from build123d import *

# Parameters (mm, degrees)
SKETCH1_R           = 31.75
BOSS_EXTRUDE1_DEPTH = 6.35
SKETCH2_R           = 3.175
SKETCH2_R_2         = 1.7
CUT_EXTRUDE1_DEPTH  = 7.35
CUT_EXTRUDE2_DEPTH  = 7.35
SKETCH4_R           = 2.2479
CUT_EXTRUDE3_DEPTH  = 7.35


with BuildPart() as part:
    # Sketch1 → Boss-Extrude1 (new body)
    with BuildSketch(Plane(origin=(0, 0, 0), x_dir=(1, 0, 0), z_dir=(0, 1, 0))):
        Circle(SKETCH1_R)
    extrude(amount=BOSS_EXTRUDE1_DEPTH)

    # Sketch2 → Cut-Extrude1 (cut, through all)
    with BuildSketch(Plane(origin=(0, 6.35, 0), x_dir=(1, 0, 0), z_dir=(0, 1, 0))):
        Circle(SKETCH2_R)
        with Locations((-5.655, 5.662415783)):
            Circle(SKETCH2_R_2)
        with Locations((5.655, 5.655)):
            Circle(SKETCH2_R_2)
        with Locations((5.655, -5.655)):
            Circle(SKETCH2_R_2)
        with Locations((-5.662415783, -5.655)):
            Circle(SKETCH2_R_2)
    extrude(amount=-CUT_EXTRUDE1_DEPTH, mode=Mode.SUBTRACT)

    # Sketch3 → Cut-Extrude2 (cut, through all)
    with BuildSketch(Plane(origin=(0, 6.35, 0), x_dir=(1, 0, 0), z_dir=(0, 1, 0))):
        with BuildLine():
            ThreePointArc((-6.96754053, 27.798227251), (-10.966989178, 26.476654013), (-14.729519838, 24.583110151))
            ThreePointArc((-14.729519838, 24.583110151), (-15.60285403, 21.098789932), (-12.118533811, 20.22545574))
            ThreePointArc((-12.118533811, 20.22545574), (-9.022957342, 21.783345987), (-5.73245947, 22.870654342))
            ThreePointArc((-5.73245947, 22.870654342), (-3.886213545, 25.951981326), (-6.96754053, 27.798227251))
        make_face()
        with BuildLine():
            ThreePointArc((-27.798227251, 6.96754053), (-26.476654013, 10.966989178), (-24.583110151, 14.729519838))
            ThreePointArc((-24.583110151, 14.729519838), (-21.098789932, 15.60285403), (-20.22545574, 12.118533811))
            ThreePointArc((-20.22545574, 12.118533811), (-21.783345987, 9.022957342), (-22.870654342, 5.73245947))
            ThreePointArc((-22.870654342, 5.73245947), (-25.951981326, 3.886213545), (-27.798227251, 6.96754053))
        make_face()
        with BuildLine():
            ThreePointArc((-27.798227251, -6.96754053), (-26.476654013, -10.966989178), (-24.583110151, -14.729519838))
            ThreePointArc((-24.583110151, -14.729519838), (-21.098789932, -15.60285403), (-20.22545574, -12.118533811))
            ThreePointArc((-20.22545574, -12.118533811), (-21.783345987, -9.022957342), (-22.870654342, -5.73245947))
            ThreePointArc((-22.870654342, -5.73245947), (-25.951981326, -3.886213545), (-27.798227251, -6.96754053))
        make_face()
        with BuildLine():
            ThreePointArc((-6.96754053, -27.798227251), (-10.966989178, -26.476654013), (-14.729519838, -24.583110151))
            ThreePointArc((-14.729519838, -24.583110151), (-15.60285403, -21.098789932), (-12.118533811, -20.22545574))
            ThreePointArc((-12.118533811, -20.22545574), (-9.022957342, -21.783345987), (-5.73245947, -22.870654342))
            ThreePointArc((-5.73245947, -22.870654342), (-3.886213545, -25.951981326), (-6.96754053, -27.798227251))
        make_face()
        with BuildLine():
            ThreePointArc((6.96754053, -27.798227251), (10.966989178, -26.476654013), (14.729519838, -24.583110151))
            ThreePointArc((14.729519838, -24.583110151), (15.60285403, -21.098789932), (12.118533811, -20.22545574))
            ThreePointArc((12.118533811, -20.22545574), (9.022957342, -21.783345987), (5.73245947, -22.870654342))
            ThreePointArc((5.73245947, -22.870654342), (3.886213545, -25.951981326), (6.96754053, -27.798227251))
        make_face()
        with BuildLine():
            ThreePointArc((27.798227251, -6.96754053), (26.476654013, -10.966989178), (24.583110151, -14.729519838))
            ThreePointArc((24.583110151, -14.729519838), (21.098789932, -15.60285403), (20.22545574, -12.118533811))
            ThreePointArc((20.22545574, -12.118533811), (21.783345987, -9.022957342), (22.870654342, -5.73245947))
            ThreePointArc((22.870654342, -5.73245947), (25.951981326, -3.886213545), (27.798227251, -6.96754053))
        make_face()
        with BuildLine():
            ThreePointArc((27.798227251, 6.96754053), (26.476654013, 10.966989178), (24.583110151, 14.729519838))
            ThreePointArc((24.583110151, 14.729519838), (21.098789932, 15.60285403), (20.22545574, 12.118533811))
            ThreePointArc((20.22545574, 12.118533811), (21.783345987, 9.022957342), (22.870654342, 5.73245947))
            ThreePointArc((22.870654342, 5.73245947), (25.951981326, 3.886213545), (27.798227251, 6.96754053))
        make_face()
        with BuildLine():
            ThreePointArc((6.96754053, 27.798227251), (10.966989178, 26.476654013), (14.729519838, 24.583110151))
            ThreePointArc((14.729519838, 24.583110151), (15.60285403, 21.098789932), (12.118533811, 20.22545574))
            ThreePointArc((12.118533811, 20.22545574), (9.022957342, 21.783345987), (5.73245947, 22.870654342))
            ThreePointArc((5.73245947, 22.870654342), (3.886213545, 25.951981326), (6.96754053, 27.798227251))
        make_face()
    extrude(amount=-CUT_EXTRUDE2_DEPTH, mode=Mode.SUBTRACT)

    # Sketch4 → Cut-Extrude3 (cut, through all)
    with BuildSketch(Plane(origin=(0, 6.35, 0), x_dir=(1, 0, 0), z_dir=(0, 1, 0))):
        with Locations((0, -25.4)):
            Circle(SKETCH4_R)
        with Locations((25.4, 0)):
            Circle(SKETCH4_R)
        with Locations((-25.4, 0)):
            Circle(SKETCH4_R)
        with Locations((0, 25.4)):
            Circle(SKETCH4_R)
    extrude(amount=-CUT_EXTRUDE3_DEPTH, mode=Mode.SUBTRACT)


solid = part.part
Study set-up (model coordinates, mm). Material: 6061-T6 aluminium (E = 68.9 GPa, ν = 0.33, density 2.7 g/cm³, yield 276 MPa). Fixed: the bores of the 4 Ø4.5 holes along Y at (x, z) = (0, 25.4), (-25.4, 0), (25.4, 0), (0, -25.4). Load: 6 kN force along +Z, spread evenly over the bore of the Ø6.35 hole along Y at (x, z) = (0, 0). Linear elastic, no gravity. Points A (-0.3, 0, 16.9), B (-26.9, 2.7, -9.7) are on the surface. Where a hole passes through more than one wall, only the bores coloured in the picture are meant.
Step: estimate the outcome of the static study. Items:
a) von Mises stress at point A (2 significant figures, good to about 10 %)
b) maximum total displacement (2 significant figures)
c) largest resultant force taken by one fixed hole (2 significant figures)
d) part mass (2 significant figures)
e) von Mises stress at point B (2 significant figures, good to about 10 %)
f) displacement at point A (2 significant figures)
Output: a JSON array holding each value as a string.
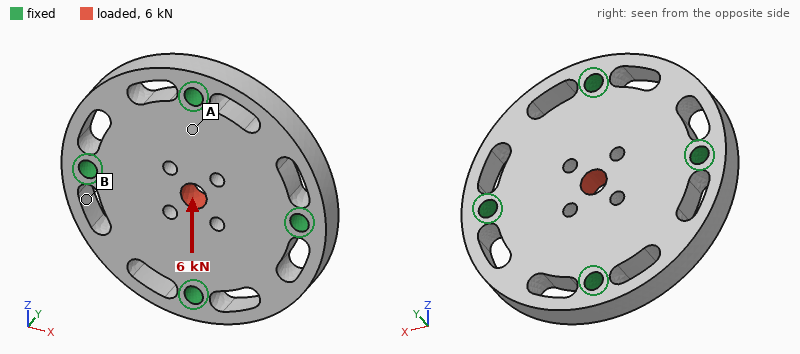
["39 MPa", "12 µm", "2.2 kN", "44 g", "10 MPa", "3.6 µm"]
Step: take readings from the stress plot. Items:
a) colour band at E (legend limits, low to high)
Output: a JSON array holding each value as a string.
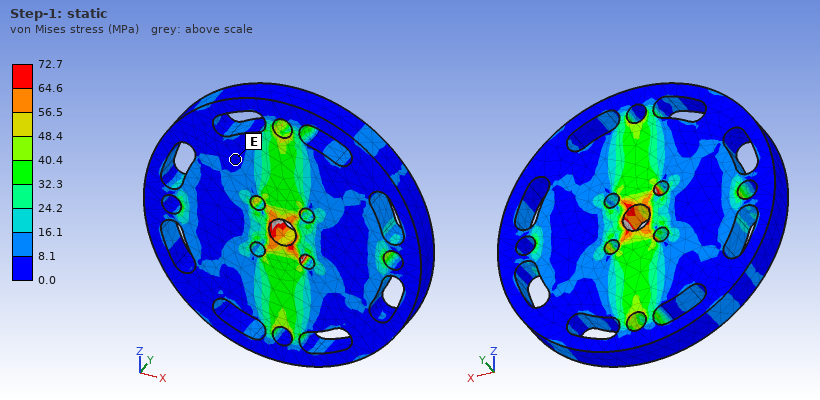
["0.0 to 8.1 MPa"]
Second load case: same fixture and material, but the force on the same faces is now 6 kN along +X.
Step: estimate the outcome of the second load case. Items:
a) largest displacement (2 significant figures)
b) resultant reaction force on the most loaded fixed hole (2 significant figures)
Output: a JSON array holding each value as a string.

["12 µm", "2.2 kN"]
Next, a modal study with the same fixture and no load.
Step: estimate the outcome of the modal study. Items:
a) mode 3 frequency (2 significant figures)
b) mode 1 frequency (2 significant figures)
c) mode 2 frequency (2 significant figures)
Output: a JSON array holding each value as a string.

["16 kHz", "15 kHz", "16 kHz"]
